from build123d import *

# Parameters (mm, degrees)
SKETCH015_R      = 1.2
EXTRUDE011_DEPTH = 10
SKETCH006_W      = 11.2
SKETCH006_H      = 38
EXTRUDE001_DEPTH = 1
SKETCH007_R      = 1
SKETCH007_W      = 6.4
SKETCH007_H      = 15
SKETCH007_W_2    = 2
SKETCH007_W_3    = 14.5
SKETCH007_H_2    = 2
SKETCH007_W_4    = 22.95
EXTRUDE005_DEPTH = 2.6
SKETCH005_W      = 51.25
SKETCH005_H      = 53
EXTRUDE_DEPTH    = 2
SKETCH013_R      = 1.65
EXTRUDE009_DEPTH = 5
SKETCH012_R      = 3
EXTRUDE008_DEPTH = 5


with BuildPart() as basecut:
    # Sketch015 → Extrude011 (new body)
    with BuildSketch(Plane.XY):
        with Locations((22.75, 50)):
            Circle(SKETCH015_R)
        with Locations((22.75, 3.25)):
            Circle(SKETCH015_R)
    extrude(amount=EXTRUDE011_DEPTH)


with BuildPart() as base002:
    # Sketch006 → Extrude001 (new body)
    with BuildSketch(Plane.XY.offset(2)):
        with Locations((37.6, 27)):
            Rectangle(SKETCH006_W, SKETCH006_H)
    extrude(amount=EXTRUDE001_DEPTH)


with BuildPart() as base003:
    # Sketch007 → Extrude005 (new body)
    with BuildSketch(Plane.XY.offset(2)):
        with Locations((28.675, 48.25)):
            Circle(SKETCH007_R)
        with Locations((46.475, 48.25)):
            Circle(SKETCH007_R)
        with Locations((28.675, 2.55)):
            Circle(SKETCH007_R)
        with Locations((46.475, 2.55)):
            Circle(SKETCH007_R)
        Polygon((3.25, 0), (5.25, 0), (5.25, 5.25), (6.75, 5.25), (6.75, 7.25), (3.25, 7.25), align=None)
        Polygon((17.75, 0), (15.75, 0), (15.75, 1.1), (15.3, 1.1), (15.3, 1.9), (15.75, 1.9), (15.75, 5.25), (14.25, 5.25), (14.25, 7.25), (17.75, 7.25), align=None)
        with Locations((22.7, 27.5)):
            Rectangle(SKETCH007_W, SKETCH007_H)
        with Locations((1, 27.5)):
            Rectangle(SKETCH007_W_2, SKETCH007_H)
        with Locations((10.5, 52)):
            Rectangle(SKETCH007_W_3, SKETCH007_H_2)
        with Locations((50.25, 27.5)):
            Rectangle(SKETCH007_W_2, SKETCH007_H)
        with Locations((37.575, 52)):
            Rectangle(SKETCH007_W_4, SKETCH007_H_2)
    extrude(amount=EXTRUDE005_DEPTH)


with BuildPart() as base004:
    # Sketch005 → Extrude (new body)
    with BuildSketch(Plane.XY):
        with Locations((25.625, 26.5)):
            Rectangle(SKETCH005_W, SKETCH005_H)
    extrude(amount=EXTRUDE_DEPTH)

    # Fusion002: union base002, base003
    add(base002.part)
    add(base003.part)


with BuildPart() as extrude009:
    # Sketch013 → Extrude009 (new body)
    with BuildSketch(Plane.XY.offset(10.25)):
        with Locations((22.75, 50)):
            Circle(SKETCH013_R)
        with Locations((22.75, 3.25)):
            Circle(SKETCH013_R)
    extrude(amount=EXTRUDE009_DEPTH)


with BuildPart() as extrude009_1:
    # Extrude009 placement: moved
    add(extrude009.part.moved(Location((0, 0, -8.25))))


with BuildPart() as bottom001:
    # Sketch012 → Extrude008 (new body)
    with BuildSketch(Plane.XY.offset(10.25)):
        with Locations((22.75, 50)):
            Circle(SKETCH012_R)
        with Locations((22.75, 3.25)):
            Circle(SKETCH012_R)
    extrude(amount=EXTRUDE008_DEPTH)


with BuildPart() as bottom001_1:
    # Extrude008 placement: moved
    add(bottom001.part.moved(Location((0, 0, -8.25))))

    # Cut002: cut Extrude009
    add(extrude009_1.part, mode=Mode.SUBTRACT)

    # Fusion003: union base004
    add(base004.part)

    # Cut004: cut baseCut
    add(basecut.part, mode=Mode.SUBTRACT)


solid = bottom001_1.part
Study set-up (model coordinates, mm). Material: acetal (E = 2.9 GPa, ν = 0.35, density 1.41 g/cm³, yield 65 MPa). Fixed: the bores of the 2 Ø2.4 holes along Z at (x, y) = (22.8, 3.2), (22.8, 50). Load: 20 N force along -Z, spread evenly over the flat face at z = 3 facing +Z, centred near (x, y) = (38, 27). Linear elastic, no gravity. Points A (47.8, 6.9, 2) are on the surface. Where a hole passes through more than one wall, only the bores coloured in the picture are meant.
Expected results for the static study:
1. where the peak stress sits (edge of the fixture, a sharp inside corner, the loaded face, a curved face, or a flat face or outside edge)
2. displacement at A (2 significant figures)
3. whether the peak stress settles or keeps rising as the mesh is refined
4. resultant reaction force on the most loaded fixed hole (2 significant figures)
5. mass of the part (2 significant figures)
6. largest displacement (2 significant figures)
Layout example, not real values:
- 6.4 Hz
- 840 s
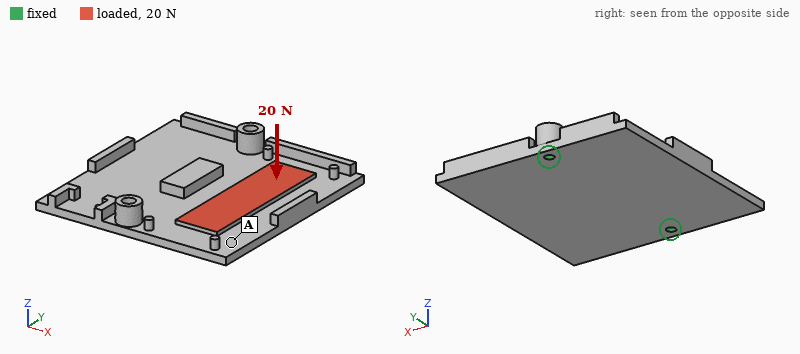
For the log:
- edge of the fixture
- 0.63 mm
- keeps rising
- 12 N
- 9.5 g
- 0.81 mm
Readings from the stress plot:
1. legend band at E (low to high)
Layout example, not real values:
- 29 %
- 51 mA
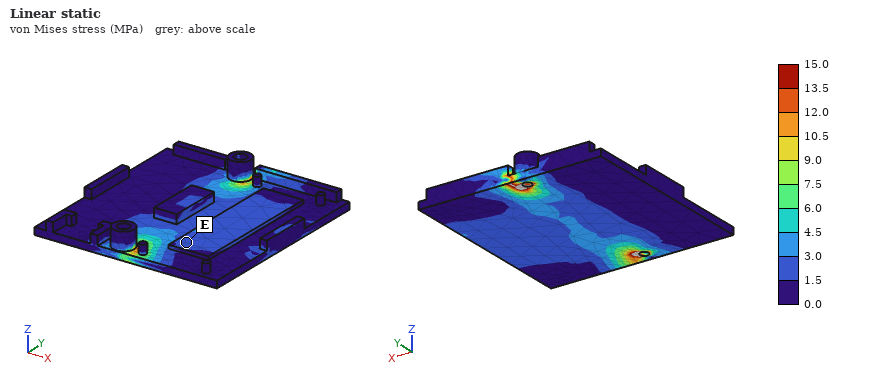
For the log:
- 1.5 to 3.0 MPa
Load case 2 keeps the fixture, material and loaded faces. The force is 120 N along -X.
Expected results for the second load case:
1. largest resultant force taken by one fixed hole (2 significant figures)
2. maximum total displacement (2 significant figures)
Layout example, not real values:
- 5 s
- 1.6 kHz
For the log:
- 61 N
- 0.76 mm
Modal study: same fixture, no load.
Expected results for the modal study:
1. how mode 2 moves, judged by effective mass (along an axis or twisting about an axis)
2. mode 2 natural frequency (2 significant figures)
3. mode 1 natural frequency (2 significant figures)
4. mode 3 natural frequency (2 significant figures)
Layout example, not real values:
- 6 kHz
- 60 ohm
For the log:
- along Z
- 730 Hz
- 420 Hz
- 1100 Hz
